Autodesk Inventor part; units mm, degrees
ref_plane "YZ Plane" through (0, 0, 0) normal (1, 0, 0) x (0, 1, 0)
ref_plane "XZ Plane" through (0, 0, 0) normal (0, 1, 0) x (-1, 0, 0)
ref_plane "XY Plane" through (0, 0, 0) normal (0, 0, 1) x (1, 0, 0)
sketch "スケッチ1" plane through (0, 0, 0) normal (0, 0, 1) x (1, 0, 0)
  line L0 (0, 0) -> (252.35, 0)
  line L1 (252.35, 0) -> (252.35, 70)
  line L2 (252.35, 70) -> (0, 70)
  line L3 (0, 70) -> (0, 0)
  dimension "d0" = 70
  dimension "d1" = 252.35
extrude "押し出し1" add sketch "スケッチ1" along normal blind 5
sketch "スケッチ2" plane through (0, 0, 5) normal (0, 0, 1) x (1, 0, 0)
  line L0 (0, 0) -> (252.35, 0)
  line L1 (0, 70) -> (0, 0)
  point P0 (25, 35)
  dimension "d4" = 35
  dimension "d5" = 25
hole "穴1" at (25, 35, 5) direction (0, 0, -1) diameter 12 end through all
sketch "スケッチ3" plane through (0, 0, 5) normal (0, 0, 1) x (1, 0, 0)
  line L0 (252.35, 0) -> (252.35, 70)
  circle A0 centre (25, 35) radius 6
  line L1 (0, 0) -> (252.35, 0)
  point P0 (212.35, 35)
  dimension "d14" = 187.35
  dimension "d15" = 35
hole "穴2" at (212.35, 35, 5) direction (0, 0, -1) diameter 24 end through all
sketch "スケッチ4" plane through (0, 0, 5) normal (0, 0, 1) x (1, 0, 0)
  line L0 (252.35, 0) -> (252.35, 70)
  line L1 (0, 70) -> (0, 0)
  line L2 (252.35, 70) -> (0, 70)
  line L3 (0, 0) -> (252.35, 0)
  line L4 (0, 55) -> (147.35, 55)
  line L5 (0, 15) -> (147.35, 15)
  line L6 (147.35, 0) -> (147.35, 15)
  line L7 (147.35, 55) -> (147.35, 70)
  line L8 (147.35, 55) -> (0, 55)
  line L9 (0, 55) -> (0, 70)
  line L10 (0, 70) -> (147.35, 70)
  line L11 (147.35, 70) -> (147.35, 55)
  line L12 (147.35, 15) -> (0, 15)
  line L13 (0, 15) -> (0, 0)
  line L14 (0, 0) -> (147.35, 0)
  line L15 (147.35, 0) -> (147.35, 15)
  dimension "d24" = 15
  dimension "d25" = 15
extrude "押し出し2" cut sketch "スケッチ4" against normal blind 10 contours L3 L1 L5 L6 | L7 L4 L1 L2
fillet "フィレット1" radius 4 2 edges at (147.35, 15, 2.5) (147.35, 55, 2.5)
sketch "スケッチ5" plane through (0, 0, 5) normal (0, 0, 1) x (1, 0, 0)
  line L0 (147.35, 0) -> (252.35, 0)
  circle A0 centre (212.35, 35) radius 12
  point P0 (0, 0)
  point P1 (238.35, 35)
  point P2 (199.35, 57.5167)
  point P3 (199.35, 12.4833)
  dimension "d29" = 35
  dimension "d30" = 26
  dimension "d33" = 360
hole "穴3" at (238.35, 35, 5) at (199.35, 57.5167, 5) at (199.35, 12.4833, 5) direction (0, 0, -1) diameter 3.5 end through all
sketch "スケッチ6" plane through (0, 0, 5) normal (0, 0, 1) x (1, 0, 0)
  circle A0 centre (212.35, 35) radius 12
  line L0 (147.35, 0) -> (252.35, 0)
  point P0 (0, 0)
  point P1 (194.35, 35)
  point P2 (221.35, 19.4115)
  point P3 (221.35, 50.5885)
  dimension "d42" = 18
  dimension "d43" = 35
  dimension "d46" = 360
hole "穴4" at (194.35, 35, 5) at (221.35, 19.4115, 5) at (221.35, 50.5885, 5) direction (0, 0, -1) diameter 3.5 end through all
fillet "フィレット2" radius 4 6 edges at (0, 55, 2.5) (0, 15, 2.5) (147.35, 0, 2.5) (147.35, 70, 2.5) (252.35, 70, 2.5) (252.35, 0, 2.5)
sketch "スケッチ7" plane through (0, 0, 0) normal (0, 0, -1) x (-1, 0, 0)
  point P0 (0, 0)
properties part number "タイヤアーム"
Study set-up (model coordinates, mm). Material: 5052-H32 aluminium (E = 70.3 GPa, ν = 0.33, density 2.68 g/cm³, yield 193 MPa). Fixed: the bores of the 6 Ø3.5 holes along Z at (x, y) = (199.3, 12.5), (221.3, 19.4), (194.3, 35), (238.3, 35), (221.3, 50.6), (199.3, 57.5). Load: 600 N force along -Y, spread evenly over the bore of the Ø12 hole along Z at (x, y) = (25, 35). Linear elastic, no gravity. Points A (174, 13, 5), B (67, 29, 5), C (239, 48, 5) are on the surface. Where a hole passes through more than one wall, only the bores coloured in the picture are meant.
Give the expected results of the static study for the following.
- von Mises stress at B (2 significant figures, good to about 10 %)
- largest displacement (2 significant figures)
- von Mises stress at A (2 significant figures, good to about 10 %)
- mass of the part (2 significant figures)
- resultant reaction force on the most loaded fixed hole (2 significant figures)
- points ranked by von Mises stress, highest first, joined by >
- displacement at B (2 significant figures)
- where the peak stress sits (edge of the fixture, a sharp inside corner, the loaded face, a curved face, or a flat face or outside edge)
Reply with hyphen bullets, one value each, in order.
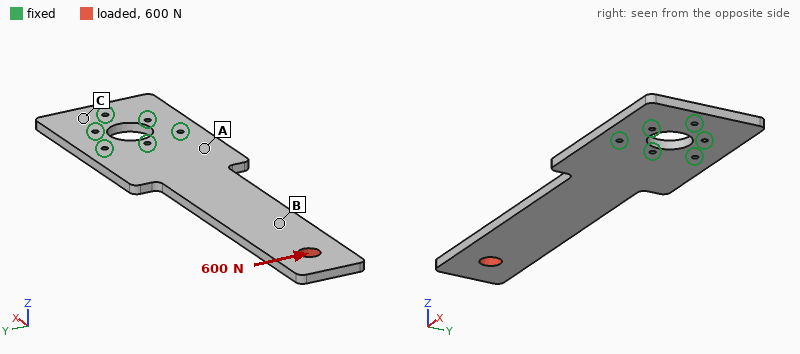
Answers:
- 9.1 MPa
- 0.41 mm
- 17 MPa
- 170 g
- 1.7 kN
- A > B > C
- 0.19 mm
- a curved face
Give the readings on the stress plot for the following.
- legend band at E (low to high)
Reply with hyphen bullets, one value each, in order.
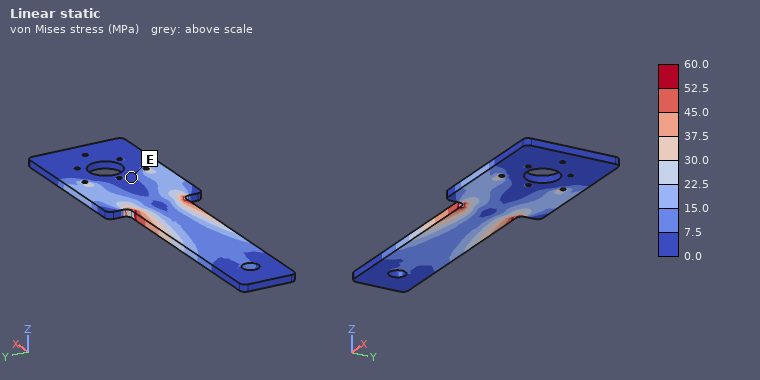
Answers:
- 0.0 to 7.5 MPa
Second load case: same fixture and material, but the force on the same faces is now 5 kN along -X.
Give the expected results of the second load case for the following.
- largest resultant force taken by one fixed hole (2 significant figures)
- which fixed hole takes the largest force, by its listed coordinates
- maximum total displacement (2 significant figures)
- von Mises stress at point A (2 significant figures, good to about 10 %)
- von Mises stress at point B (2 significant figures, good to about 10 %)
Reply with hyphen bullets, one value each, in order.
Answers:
- 1.6 kN
- (194.3, 35)
- 64 µm
- 14 MPa
- 25 MPa
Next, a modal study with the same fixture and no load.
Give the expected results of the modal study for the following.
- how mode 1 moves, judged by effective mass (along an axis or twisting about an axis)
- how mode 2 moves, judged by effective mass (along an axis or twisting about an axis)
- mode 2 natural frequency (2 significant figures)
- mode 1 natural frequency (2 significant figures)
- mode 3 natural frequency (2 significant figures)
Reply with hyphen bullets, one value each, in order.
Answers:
- along Z
- along Z
- 720 Hz
- 130 Hz
- 1100 Hz
